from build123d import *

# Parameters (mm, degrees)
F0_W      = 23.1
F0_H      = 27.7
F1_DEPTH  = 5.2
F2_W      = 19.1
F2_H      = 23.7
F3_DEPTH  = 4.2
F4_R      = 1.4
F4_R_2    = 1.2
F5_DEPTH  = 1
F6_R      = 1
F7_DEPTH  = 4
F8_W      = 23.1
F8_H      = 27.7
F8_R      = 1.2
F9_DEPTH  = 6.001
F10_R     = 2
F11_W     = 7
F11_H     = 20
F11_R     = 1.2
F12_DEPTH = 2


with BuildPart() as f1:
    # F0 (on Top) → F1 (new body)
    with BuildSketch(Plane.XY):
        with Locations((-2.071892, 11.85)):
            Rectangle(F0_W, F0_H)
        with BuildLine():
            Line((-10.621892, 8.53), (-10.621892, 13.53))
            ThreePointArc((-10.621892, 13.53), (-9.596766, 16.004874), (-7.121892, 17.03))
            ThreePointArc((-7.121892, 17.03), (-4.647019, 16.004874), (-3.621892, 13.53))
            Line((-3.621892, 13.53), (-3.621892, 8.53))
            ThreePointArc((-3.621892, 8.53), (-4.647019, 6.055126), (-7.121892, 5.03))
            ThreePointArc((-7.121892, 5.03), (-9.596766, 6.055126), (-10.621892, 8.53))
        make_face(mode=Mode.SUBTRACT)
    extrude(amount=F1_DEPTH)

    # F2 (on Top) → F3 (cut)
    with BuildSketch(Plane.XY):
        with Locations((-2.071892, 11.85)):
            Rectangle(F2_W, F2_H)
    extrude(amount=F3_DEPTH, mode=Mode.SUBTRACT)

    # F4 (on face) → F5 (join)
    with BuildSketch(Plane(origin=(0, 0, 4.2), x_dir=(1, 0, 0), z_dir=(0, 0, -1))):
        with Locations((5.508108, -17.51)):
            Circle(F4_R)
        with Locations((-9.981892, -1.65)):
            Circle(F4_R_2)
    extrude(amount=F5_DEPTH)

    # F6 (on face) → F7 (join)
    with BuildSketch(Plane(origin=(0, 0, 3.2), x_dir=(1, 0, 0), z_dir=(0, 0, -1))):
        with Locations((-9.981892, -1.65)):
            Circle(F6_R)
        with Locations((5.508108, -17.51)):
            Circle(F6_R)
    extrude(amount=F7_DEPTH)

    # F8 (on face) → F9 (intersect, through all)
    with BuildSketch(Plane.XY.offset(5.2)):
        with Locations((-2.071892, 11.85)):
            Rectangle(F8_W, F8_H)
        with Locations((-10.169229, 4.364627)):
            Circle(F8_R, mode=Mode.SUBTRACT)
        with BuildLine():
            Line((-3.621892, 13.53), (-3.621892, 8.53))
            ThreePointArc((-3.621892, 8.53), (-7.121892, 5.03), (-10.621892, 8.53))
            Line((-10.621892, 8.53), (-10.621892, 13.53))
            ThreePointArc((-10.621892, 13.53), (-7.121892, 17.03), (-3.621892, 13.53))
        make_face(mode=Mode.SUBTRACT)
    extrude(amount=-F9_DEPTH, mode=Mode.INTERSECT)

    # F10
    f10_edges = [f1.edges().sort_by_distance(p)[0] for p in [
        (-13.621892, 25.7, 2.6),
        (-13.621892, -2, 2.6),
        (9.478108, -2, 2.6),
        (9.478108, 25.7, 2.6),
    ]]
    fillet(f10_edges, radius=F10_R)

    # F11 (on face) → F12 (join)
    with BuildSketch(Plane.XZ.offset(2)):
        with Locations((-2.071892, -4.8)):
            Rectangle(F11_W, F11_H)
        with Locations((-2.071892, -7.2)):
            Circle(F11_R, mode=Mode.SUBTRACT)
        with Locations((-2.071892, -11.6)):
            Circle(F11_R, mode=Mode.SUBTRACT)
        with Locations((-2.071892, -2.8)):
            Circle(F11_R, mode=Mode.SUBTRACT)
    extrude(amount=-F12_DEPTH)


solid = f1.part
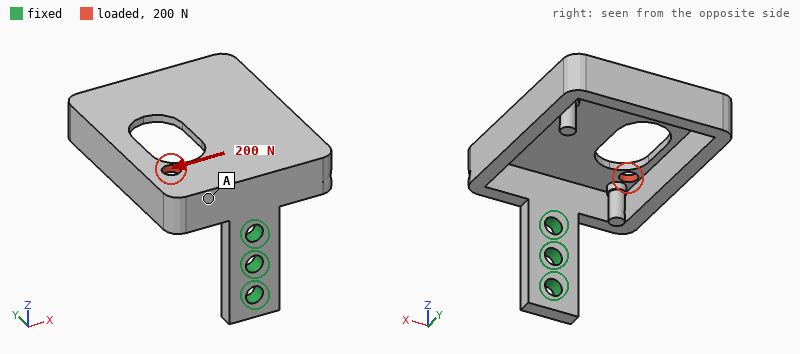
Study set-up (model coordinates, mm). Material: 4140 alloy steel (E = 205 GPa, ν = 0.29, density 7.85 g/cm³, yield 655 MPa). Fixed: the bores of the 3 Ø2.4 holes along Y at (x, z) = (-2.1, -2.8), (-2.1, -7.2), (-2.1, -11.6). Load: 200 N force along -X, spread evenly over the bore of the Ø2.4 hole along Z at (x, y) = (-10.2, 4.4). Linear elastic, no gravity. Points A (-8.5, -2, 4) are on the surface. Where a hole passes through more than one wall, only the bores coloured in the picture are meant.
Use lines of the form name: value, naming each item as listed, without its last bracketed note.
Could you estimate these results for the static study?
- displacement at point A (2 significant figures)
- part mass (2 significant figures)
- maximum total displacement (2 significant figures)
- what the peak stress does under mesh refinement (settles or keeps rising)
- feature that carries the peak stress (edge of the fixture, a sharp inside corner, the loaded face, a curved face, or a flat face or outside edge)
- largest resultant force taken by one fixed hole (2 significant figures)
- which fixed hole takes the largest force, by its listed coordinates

displacement at point A: 0.022 mm
part mass: 12 g
maximum total displacement: 0.11 mm
what the peak stress does under mesh refinement: keeps rising
feature that carries the peak stress: edge of the fixture
largest resultant force taken by one fixed hole: 310 N
which fixed hole takes the largest force, by its listed coordinates: (-2.1, -2.8)
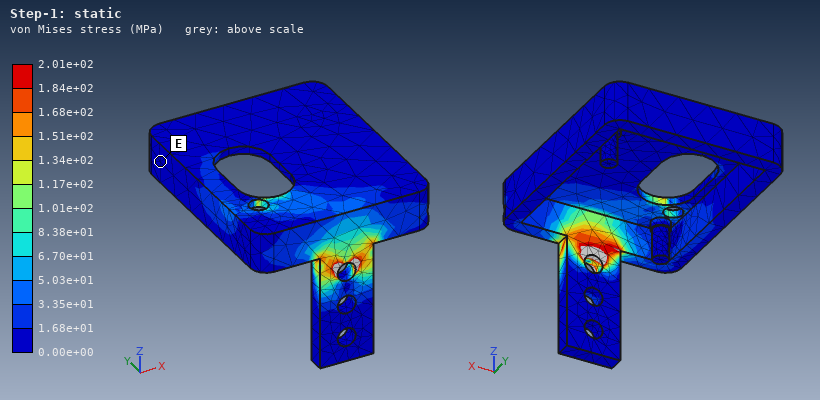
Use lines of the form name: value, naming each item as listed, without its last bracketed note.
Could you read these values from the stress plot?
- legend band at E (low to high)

legend band at E: 0.00e+00 to 1.68e+01 MPa
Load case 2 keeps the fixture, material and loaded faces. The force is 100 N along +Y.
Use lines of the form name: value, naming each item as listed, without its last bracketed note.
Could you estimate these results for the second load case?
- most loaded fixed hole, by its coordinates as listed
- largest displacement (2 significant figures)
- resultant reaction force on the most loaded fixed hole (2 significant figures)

most loaded fixed hole, by its coordinates as listed: (-2.1, -2.8)
largest displacement: 0.10 mm
resultant reaction force on the most loaded fixed hole: 120 N
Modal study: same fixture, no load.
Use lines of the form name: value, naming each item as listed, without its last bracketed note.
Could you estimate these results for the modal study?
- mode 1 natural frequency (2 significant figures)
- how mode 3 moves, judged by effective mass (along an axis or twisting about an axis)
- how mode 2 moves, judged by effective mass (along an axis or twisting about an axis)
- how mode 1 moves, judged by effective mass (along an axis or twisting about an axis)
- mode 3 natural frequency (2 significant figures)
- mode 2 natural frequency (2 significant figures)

mode 1 natural frequency: 1100 Hz
how mode 3 moves, judged by effective mass: twisting about Y
how mode 2 moves, judged by effective mass: along X
how mode 1 moves, judged by effective mass: along Z
mode 3 natural frequency: 3600 Hz
mode 2 natural frequency: 1500 Hz
